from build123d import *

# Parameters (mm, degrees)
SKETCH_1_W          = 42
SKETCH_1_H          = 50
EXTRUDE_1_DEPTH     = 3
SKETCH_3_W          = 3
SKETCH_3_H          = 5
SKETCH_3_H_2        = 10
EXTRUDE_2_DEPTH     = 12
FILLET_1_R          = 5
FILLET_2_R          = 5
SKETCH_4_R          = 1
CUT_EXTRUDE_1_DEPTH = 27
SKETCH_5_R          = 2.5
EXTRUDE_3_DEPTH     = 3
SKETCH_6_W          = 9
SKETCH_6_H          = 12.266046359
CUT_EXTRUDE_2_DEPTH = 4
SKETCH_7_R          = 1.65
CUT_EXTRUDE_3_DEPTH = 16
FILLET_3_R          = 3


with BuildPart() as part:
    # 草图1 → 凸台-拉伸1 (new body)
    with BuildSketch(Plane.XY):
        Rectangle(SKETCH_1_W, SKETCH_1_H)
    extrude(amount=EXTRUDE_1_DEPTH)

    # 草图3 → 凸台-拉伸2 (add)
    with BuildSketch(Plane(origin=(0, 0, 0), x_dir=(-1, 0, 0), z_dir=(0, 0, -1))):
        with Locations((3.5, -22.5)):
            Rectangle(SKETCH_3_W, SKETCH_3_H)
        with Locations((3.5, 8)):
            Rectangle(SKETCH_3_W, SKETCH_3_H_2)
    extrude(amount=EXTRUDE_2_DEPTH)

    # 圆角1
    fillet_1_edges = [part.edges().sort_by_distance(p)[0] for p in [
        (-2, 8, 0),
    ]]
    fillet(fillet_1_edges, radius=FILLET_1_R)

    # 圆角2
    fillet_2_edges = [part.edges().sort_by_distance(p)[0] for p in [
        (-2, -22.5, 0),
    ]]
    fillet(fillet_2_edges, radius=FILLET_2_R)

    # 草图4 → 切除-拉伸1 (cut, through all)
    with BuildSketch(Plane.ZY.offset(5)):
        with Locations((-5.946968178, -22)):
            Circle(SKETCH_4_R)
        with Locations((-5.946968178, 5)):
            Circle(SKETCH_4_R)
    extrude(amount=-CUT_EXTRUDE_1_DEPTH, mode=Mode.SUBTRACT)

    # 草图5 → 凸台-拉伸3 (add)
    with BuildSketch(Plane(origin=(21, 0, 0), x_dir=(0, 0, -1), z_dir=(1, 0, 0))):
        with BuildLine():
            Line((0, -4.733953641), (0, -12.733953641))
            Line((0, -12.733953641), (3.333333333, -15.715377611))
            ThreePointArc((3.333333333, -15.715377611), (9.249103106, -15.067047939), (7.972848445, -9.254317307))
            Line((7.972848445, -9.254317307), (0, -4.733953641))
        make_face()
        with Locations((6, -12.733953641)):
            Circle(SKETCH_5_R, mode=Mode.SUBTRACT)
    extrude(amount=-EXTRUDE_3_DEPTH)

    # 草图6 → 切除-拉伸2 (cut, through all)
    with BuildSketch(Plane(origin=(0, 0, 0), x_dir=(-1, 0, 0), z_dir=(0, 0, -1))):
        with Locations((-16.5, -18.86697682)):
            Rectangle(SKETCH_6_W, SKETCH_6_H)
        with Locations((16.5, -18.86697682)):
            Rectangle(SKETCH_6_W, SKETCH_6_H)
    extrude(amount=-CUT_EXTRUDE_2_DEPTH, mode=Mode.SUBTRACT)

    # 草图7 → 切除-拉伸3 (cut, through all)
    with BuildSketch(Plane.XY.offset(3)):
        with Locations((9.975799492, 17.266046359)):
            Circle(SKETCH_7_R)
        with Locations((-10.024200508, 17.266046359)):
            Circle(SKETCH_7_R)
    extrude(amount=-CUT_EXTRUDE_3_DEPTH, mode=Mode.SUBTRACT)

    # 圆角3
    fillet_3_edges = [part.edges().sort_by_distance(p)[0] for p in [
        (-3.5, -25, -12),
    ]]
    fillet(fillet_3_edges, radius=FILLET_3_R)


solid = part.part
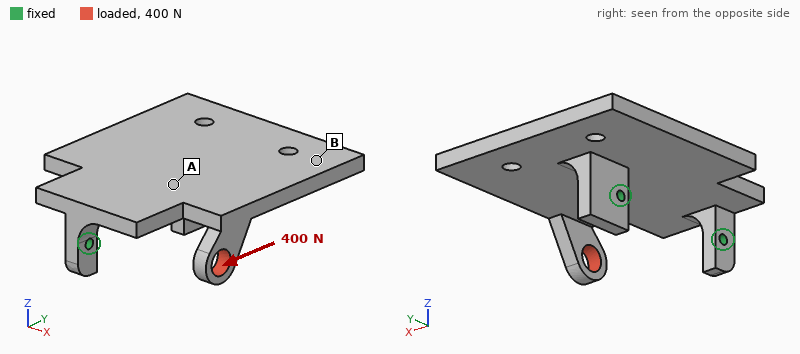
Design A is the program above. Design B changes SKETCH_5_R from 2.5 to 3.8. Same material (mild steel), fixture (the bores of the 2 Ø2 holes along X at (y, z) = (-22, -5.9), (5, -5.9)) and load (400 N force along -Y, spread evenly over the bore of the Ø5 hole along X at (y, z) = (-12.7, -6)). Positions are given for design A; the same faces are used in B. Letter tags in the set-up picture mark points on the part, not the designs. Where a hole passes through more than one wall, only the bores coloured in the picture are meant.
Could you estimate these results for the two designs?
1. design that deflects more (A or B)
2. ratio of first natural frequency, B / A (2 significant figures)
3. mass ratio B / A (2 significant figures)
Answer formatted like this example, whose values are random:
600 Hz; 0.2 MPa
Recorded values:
B; 1.0; 0.99
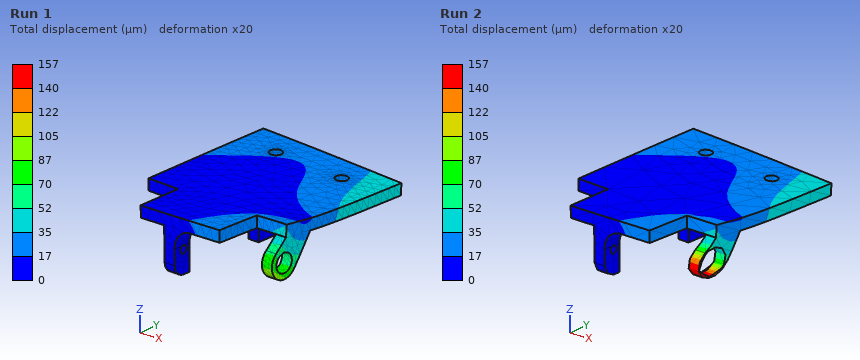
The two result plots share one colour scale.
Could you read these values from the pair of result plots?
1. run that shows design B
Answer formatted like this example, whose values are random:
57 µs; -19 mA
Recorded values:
Run 2
